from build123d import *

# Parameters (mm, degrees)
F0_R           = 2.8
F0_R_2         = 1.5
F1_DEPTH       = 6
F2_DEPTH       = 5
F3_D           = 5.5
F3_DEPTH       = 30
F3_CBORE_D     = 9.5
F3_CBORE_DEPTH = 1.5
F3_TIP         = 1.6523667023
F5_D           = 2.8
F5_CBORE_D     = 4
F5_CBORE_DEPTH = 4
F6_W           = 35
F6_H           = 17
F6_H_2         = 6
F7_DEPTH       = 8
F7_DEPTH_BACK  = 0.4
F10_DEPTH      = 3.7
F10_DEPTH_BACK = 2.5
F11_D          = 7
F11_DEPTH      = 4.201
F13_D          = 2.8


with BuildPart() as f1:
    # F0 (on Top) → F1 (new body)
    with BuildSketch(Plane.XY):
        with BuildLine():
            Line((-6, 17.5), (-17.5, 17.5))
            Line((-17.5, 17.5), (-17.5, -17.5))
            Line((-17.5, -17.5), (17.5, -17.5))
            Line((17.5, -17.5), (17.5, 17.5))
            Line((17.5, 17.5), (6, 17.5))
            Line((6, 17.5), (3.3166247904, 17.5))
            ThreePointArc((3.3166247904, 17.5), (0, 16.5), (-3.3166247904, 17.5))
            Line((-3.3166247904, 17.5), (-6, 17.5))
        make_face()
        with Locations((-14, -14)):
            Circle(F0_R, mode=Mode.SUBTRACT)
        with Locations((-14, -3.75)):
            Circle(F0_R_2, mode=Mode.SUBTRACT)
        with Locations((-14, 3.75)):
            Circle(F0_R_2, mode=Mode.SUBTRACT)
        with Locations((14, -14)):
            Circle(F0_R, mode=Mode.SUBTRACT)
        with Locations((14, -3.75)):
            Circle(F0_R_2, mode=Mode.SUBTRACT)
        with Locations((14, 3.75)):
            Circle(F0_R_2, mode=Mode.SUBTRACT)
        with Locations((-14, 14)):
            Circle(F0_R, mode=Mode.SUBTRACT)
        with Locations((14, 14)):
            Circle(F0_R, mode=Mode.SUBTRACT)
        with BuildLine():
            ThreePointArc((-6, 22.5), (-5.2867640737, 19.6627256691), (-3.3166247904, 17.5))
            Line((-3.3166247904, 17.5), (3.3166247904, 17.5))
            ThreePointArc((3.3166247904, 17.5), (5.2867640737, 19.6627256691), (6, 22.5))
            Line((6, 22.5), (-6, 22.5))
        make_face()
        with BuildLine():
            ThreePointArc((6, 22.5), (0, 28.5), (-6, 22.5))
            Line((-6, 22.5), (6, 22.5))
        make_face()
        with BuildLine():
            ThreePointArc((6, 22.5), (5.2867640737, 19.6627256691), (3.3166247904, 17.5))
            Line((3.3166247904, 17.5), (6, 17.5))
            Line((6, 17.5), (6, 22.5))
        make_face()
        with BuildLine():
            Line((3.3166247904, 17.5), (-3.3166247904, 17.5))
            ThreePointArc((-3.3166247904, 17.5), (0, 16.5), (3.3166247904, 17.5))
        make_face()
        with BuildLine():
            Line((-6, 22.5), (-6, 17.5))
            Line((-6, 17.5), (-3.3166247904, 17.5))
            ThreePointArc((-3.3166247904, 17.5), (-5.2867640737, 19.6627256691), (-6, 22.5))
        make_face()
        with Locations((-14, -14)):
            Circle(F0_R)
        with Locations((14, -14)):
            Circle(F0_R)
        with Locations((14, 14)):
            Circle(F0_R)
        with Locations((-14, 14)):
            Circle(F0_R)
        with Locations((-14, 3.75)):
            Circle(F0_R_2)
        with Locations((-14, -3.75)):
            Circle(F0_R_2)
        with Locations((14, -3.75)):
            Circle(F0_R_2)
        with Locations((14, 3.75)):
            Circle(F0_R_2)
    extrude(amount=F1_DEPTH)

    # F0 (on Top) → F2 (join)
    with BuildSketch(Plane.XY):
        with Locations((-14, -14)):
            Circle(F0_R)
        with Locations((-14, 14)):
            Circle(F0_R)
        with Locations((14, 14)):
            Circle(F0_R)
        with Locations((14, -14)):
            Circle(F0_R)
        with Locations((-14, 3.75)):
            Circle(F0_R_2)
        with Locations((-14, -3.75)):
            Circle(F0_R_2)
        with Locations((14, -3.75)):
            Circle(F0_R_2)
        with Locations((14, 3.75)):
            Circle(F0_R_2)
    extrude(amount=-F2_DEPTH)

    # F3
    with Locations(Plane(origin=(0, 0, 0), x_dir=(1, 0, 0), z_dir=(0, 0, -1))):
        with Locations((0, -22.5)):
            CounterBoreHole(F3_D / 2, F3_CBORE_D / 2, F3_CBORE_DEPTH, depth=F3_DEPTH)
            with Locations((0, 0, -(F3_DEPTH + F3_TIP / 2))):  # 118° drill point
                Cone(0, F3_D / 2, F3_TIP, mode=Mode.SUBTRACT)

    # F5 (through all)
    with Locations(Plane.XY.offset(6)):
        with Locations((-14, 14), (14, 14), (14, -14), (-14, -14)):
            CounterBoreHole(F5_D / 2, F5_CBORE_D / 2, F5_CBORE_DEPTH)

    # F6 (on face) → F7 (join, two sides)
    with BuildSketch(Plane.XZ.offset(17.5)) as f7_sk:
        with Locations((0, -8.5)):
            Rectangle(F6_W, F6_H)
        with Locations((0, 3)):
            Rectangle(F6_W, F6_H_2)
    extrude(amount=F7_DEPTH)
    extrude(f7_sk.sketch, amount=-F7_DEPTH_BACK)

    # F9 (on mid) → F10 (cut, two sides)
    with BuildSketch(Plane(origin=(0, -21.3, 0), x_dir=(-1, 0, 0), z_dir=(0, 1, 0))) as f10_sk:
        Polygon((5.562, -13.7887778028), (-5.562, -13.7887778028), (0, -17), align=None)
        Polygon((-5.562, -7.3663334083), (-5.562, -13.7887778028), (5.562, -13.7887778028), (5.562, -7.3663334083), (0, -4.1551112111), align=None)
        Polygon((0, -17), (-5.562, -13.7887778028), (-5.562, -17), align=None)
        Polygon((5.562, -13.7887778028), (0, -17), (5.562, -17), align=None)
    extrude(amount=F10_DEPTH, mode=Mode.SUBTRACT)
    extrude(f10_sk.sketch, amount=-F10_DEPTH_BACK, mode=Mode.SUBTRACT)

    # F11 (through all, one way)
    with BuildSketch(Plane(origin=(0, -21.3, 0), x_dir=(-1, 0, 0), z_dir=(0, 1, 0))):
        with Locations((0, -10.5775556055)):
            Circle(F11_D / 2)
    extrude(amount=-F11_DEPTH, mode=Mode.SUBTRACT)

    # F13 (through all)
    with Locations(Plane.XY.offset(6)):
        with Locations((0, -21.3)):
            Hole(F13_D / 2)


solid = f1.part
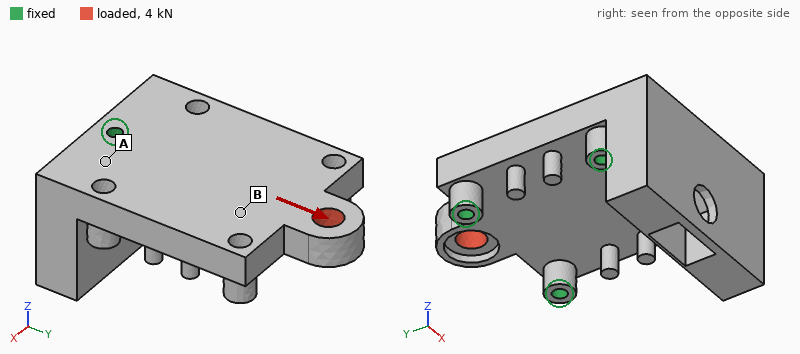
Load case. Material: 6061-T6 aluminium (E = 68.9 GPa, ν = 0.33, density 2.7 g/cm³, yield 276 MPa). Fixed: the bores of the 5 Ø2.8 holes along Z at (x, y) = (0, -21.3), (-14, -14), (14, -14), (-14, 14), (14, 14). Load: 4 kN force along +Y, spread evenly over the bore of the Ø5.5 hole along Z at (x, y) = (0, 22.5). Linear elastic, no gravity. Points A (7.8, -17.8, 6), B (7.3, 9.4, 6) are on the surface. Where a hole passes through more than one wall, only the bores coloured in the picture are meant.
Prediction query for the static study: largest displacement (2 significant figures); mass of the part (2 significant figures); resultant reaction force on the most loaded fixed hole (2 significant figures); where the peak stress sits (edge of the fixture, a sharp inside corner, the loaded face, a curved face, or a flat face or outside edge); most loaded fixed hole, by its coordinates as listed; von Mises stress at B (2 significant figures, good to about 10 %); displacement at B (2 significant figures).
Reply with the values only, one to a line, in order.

45 µm
37 g
940 N
edge of the fixture
(0, -21.3)
44 MPa
7.6 µm
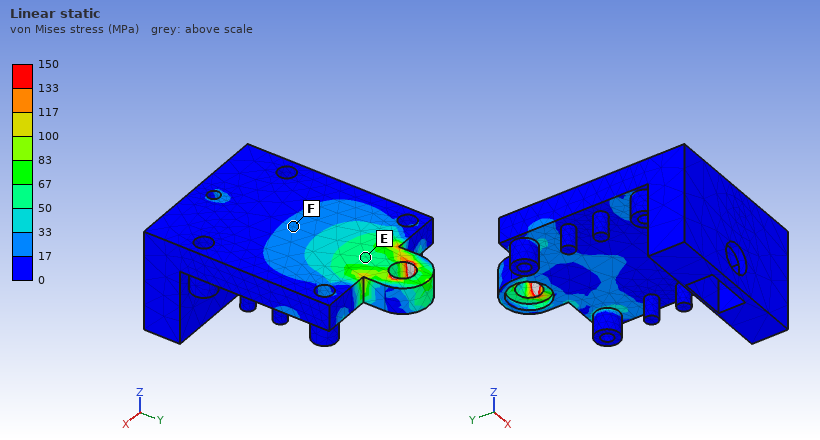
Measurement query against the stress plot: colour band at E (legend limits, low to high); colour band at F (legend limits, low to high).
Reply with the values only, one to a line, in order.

50 to 67 MPa
17 to 33 MPa
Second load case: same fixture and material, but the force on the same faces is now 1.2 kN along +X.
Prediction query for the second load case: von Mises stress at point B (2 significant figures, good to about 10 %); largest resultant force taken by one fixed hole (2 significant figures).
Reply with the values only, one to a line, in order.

11 MPa
630 N
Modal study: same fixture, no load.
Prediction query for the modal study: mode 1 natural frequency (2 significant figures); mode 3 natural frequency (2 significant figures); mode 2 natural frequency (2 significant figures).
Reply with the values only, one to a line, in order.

15 kHz
16 kHz
15 kHz
